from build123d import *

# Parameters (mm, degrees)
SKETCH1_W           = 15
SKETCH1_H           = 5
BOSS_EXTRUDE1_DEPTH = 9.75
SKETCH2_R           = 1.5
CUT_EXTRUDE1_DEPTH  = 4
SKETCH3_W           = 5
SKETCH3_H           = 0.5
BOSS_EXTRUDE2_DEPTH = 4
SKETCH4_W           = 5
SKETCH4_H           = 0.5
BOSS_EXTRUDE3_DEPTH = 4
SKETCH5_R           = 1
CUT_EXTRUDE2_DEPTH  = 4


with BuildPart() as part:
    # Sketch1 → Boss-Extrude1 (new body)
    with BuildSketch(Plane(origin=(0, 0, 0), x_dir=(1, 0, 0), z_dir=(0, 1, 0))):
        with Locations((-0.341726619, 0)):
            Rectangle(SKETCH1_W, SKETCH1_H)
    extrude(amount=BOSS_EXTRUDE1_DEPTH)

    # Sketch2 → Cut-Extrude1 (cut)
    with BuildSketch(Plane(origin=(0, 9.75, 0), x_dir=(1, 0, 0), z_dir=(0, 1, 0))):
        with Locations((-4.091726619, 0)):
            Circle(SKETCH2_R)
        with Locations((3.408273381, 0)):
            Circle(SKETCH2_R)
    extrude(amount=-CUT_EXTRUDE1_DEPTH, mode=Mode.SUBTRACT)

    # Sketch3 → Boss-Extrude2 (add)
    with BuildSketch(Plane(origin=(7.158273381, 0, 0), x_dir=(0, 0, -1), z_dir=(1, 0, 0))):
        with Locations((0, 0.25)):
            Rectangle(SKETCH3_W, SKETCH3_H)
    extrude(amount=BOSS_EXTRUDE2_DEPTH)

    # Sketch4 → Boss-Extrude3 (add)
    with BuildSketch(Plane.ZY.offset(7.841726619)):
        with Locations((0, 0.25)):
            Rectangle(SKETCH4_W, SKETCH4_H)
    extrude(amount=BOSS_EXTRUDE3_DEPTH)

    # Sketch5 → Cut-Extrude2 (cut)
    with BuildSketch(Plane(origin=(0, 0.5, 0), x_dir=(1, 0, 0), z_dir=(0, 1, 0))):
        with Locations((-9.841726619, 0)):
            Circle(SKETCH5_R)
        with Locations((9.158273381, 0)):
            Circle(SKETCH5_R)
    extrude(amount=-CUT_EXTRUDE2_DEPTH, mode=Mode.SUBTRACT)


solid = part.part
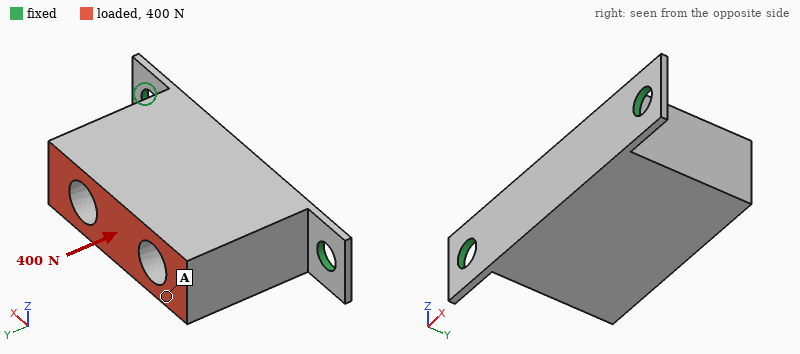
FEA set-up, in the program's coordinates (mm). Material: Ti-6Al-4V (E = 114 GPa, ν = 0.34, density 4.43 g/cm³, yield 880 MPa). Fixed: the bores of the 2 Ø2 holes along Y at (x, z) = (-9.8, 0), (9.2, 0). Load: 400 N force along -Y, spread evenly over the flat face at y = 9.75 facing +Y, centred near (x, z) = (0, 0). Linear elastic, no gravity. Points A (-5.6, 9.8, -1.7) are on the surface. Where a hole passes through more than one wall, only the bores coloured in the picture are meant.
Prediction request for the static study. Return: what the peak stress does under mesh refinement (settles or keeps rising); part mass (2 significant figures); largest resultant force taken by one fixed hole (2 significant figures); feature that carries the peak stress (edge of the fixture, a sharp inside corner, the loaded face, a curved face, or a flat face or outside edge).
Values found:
keeps rising
3.1 g
230 N
edge of the fixture
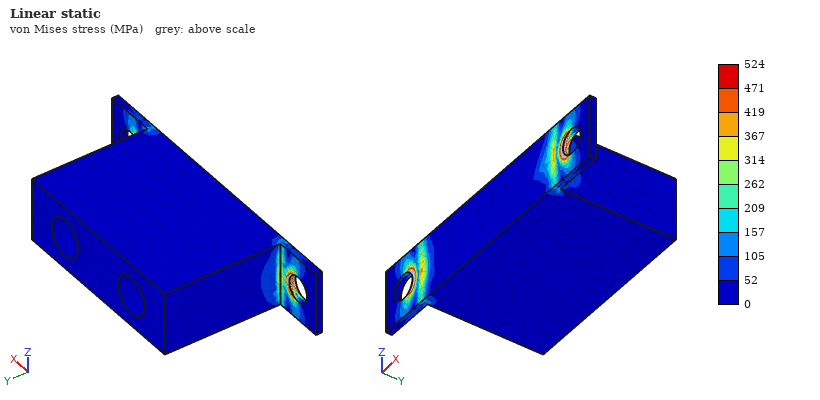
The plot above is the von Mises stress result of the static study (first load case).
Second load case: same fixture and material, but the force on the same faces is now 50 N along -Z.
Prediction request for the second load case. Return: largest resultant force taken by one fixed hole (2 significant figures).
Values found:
25 N
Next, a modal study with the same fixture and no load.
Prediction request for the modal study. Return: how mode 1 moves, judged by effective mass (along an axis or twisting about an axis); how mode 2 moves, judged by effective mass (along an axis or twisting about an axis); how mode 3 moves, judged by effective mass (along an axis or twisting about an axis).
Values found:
along Z
along Y
along X
